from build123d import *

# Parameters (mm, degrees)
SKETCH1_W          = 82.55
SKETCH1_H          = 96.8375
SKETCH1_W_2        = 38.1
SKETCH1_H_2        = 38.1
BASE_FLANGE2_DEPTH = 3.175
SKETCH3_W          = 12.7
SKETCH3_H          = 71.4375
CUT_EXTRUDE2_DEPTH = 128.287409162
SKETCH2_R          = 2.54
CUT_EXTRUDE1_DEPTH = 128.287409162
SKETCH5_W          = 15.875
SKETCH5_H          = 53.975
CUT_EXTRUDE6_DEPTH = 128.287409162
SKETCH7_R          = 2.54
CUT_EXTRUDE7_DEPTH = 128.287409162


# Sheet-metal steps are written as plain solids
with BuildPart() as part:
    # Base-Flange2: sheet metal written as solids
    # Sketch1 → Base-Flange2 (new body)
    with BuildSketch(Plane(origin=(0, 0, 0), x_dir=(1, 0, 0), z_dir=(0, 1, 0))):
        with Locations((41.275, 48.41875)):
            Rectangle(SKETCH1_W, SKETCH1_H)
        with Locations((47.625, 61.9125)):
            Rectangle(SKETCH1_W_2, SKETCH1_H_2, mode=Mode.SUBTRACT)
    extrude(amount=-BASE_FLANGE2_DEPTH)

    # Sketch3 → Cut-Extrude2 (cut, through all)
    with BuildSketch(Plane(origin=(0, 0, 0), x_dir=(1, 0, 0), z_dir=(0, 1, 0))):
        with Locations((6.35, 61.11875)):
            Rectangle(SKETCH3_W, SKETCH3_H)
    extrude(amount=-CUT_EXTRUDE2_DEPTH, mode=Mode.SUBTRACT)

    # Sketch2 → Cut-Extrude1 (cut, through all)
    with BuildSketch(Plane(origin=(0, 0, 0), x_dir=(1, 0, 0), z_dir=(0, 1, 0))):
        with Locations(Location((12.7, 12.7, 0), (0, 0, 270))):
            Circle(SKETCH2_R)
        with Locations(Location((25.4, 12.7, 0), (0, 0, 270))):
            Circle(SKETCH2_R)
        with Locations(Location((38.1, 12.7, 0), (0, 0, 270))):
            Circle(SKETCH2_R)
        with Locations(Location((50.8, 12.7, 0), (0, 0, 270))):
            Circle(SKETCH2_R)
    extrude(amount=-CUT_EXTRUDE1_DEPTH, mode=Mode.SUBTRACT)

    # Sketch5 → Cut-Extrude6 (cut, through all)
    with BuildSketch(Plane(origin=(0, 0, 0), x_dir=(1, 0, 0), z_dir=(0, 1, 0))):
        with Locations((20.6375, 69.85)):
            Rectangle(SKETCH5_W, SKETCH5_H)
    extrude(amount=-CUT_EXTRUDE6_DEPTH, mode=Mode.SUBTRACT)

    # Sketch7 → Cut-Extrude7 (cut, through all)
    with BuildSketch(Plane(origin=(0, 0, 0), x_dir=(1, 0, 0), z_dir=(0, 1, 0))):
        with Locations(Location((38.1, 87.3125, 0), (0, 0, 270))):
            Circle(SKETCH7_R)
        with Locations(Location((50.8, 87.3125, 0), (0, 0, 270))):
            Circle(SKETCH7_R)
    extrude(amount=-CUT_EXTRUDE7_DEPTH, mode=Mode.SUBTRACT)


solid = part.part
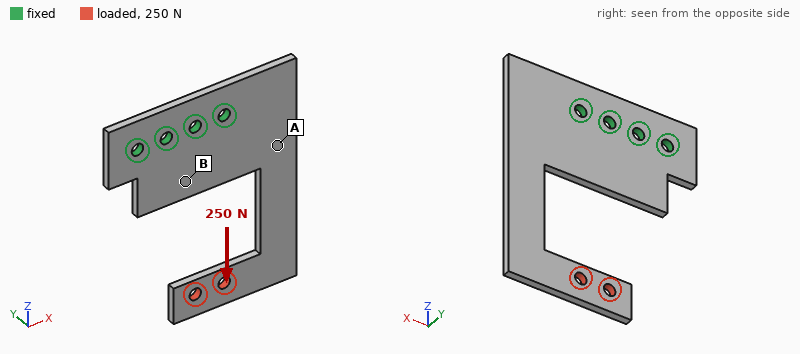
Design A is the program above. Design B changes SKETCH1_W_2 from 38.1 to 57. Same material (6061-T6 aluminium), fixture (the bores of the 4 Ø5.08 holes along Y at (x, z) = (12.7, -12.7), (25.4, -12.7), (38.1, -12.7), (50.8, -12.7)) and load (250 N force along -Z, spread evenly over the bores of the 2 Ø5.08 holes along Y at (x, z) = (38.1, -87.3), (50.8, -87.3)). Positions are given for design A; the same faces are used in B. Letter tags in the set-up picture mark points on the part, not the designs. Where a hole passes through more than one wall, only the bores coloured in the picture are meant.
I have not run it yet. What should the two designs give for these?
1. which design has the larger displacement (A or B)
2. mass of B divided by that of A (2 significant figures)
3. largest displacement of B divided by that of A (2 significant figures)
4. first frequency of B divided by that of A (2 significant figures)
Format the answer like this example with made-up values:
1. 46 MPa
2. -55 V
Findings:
1. B
2. 0.92
3. 14
4. 0.71
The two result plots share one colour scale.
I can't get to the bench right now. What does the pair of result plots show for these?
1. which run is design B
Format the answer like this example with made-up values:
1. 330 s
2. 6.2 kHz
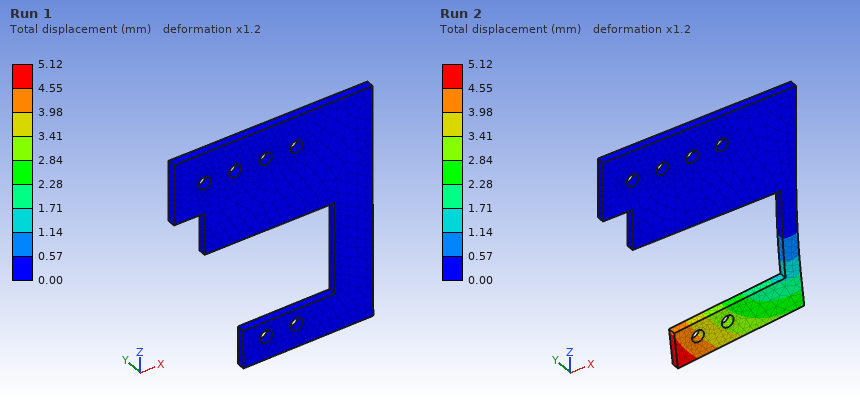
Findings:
1. Run 2
